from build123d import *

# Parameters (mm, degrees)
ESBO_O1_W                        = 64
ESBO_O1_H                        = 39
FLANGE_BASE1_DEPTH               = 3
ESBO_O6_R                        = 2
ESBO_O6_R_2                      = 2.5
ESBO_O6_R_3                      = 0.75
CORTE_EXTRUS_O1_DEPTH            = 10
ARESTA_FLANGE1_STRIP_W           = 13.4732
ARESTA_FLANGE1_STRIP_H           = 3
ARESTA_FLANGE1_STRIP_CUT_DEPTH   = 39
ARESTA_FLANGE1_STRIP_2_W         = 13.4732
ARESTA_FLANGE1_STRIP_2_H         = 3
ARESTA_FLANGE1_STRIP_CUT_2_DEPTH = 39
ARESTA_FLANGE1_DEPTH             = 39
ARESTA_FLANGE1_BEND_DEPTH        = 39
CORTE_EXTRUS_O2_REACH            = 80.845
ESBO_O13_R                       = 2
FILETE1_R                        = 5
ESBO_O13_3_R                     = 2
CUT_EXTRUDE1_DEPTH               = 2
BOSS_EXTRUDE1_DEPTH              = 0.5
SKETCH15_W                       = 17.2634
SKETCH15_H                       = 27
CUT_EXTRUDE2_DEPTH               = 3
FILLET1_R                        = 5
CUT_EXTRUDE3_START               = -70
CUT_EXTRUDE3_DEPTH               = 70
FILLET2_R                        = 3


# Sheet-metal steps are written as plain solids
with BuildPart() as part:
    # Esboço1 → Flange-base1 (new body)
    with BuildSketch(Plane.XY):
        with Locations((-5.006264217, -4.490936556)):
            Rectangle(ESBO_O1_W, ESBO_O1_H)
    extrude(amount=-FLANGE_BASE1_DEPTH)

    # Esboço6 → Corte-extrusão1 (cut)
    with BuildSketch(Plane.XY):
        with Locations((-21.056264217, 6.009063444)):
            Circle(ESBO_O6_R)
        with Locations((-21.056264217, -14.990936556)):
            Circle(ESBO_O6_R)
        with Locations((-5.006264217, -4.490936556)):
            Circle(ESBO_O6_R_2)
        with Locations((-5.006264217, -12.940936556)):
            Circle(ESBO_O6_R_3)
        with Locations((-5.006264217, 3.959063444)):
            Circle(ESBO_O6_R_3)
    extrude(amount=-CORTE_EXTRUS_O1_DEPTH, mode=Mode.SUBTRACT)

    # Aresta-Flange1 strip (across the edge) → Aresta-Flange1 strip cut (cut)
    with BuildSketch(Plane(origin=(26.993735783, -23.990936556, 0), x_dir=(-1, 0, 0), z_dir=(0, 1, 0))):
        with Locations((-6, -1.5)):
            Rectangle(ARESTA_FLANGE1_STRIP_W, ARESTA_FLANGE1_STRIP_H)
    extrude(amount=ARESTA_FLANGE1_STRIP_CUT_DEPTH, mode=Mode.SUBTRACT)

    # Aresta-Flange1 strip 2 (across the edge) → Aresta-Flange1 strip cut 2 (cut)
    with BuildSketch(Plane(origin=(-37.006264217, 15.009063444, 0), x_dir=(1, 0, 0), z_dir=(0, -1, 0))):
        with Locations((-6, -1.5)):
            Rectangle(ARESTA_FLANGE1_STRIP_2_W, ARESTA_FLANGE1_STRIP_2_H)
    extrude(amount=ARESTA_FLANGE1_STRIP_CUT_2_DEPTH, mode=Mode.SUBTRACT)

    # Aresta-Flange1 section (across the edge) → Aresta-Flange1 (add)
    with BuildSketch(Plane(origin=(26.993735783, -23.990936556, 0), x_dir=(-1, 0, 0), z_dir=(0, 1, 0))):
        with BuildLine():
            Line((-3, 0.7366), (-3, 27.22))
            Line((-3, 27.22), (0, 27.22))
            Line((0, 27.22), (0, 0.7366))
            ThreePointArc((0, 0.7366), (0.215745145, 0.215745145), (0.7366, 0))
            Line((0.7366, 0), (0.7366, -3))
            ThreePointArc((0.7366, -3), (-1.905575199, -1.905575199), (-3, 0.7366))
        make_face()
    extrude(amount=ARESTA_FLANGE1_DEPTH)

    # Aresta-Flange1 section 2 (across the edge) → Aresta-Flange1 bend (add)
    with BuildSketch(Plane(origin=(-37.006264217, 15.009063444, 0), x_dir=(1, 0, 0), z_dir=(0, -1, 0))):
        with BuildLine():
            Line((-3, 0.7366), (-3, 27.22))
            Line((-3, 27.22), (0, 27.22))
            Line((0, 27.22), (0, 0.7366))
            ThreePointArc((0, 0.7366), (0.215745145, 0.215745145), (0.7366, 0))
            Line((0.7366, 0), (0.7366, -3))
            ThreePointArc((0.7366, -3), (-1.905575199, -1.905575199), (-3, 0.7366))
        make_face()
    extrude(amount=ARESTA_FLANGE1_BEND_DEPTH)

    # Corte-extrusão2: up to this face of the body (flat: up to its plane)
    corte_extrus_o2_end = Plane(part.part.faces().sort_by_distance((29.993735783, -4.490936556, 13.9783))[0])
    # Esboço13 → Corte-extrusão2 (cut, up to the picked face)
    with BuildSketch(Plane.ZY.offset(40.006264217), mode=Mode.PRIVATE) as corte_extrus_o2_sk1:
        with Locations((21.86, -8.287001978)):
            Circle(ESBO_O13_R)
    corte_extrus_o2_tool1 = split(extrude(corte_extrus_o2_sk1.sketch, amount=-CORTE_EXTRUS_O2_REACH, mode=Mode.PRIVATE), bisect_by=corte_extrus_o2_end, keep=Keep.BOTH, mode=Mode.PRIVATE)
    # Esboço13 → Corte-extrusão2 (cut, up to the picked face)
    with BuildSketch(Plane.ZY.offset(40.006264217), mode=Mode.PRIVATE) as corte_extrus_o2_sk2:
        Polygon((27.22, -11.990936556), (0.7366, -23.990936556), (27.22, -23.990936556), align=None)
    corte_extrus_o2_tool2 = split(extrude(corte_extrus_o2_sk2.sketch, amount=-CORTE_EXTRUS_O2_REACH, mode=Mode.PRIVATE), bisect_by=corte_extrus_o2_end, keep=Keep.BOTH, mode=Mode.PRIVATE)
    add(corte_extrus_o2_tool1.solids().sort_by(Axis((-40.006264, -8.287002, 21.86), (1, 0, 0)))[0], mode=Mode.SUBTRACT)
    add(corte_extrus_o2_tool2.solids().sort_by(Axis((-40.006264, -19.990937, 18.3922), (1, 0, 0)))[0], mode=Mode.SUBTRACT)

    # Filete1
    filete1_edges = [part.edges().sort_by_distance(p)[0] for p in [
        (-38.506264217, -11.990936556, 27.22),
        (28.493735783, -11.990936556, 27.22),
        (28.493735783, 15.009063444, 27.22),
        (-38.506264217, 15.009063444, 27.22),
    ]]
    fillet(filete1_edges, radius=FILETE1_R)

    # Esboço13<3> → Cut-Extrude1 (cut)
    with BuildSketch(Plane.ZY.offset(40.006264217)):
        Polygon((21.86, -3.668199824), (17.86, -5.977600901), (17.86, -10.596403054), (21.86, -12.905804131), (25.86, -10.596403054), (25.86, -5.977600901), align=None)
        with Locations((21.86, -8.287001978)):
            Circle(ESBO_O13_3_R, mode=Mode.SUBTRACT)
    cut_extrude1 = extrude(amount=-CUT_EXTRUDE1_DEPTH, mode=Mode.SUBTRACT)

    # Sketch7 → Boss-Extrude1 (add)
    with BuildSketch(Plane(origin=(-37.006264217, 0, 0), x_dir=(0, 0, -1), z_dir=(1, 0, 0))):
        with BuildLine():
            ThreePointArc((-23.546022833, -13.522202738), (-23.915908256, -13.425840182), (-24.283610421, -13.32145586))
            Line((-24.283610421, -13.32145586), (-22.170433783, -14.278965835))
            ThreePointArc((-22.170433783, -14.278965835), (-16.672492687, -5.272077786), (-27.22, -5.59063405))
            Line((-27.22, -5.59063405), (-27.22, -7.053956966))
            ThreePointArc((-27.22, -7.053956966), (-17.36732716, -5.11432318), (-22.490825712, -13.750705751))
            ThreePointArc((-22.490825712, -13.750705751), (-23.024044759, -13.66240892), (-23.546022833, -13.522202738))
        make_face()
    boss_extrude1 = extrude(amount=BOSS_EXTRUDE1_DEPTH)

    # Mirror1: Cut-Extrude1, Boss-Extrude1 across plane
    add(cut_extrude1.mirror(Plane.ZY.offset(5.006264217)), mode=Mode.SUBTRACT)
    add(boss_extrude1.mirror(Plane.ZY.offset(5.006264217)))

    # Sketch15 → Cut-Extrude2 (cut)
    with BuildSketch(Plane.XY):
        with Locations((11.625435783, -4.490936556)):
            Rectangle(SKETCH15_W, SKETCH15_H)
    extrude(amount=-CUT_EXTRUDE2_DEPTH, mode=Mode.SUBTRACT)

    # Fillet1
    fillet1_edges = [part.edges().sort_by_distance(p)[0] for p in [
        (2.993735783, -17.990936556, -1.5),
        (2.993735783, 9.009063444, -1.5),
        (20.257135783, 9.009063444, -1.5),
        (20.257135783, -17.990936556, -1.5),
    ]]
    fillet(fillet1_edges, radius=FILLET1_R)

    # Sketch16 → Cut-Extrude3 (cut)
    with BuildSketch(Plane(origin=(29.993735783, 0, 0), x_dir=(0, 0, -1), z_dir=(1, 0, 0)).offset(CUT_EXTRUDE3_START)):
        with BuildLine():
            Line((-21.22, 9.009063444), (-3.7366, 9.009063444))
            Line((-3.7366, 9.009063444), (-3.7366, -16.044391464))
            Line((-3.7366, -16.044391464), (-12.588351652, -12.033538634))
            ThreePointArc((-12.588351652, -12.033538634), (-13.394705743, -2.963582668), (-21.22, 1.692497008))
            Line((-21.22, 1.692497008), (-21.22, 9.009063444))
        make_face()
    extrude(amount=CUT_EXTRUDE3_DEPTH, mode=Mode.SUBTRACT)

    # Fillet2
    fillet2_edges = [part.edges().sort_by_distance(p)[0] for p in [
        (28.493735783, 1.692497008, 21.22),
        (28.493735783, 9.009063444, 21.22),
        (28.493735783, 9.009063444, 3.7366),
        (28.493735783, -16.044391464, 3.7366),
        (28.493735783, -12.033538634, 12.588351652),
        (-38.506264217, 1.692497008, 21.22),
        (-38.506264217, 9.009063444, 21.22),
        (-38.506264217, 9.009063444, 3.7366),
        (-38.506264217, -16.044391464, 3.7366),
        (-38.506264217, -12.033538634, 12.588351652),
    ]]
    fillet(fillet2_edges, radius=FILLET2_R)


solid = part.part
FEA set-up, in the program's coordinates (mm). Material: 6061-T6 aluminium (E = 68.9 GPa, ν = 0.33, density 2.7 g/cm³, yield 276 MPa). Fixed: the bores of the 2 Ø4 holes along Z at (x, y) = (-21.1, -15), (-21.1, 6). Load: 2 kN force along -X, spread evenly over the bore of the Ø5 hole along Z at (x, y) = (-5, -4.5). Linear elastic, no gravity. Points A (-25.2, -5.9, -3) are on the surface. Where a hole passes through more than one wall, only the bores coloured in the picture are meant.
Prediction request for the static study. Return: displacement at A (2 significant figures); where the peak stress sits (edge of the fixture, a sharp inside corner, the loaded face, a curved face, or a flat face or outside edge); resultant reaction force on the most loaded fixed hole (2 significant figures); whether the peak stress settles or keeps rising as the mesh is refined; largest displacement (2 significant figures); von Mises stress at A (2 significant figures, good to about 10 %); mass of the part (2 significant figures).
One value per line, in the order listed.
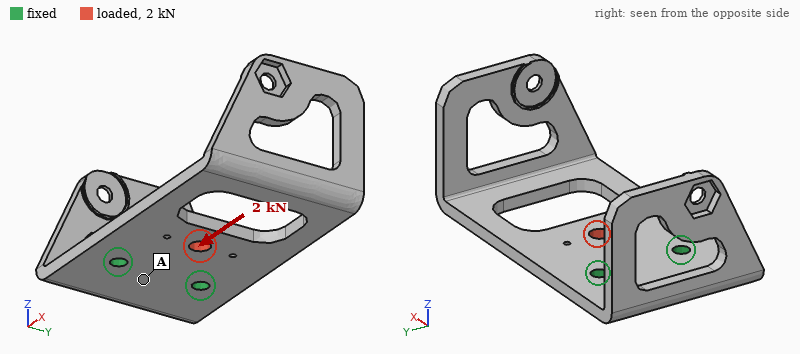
2.1 µm
a sharp inside corner
1.0 kN
keeps rising
12 µm
9.3 MPa
27 g
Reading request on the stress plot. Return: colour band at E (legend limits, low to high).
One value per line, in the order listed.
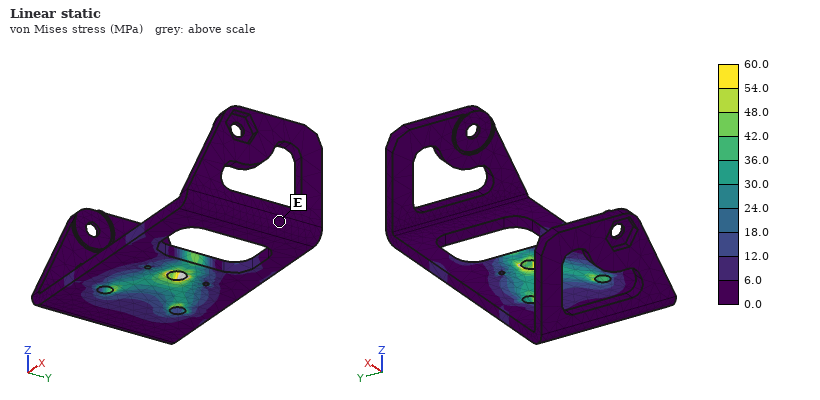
0.0 to 6.0 MPa
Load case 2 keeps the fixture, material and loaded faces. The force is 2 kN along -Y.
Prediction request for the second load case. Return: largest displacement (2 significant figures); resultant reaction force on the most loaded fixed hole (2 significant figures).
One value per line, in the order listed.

40 µm
1.7 kN
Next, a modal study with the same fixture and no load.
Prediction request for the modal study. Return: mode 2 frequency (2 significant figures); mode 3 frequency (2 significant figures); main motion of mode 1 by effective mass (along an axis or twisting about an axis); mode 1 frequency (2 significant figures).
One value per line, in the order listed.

1200 Hz
1700 Hz
along Z
540 Hz
